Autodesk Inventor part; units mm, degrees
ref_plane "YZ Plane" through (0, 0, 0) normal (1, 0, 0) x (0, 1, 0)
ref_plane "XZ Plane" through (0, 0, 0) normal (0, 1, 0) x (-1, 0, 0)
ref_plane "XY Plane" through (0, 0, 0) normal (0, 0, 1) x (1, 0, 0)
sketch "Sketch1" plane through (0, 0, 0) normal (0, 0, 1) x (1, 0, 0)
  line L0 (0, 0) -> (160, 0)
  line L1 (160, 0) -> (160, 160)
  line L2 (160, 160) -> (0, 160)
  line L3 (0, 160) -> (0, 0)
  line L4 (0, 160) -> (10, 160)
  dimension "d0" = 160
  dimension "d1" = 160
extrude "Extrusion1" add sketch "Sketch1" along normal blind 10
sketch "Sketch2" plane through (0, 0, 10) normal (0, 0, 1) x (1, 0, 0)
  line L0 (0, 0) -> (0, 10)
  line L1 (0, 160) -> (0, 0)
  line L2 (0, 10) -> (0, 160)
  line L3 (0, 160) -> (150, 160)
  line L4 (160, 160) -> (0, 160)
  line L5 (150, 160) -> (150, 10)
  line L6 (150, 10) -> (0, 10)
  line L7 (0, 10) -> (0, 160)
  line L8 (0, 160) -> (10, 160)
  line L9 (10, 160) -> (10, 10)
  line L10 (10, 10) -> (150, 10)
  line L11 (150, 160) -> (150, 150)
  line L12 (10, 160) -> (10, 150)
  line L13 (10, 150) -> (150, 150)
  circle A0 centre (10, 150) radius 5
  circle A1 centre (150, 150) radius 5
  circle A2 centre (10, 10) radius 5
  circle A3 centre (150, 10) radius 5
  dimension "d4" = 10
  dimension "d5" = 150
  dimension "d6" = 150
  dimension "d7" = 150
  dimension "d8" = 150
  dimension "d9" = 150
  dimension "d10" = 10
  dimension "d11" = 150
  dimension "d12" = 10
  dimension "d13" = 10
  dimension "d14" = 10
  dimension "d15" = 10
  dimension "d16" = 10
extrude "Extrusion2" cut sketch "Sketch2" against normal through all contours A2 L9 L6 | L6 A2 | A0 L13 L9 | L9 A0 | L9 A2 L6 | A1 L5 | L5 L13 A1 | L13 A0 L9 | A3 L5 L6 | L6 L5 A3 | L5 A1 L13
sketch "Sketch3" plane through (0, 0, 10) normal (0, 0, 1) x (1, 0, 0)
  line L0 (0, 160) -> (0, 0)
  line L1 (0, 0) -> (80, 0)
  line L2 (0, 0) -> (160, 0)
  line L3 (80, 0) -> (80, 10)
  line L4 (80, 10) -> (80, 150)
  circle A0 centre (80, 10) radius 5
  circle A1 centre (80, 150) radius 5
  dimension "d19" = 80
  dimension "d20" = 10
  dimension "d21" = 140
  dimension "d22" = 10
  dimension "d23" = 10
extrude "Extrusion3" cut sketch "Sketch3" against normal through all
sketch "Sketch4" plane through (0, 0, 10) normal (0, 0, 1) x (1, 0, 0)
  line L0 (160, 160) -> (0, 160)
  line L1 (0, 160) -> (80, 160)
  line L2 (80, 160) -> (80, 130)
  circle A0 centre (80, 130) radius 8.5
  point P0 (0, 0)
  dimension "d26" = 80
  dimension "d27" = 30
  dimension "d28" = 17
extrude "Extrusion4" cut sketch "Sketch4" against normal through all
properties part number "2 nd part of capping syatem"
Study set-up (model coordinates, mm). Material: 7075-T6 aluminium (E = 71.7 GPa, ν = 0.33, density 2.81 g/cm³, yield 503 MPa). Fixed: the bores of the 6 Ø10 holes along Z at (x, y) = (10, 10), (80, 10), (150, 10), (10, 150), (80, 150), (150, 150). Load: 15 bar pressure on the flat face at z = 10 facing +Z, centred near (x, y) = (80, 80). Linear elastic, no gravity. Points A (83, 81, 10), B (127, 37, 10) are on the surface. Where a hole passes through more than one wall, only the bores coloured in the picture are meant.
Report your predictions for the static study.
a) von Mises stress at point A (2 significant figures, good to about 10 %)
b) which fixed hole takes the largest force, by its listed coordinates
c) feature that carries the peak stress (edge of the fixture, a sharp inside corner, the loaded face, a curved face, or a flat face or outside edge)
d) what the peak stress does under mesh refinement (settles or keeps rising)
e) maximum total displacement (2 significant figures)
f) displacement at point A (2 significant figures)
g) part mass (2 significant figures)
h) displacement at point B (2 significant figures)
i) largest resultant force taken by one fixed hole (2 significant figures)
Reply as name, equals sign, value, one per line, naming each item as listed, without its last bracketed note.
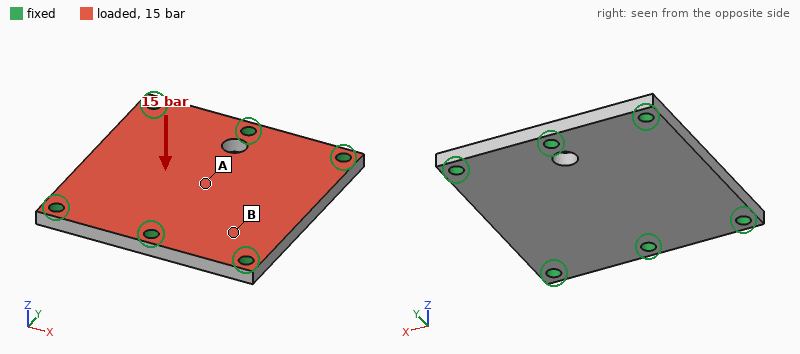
von Mises stress at point A = 73 MPa
which fixed hole takes the largest force, by its listed coordinates = (80, 10)
feature that carries the peak stress = edge of the fixture
what the peak stress does under mesh refinement = keeps rising
maximum total displacement = 0.31 mm
displacement at point A = 0.31 mm
part mass = 700 g
displacement at point B = 0.14 mm
largest resultant force taken by one fixed hole = 8.6 kN
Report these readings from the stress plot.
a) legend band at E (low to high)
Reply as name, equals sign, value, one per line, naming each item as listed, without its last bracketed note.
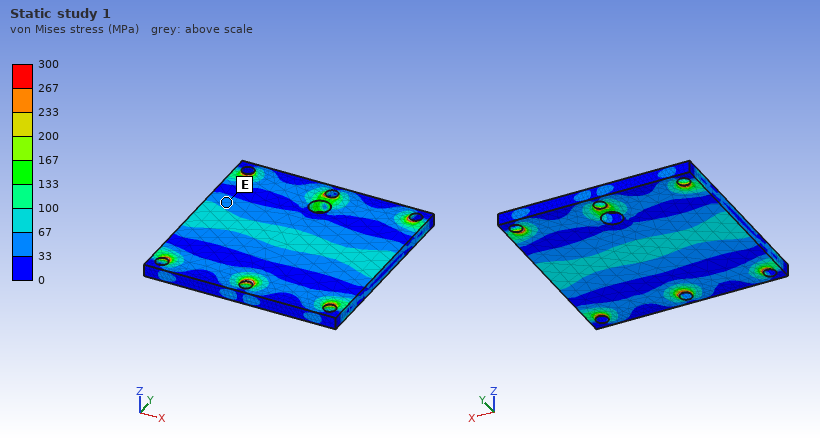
legend band at E = 33 to 67 MPa
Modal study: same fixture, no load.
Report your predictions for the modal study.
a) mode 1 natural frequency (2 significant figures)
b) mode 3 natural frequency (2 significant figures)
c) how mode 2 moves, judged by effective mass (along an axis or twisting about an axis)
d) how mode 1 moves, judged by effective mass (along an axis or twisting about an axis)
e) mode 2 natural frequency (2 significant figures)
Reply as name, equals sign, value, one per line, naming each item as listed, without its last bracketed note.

mode 1 natural frequency = 2400 Hz
mode 3 natural frequency = 4500 Hz
how mode 2 moves, judged by effective mass = twisting about Y
how mode 1 moves, judged by effective mass = along Z
mode 2 natural frequency = 2900 Hz
